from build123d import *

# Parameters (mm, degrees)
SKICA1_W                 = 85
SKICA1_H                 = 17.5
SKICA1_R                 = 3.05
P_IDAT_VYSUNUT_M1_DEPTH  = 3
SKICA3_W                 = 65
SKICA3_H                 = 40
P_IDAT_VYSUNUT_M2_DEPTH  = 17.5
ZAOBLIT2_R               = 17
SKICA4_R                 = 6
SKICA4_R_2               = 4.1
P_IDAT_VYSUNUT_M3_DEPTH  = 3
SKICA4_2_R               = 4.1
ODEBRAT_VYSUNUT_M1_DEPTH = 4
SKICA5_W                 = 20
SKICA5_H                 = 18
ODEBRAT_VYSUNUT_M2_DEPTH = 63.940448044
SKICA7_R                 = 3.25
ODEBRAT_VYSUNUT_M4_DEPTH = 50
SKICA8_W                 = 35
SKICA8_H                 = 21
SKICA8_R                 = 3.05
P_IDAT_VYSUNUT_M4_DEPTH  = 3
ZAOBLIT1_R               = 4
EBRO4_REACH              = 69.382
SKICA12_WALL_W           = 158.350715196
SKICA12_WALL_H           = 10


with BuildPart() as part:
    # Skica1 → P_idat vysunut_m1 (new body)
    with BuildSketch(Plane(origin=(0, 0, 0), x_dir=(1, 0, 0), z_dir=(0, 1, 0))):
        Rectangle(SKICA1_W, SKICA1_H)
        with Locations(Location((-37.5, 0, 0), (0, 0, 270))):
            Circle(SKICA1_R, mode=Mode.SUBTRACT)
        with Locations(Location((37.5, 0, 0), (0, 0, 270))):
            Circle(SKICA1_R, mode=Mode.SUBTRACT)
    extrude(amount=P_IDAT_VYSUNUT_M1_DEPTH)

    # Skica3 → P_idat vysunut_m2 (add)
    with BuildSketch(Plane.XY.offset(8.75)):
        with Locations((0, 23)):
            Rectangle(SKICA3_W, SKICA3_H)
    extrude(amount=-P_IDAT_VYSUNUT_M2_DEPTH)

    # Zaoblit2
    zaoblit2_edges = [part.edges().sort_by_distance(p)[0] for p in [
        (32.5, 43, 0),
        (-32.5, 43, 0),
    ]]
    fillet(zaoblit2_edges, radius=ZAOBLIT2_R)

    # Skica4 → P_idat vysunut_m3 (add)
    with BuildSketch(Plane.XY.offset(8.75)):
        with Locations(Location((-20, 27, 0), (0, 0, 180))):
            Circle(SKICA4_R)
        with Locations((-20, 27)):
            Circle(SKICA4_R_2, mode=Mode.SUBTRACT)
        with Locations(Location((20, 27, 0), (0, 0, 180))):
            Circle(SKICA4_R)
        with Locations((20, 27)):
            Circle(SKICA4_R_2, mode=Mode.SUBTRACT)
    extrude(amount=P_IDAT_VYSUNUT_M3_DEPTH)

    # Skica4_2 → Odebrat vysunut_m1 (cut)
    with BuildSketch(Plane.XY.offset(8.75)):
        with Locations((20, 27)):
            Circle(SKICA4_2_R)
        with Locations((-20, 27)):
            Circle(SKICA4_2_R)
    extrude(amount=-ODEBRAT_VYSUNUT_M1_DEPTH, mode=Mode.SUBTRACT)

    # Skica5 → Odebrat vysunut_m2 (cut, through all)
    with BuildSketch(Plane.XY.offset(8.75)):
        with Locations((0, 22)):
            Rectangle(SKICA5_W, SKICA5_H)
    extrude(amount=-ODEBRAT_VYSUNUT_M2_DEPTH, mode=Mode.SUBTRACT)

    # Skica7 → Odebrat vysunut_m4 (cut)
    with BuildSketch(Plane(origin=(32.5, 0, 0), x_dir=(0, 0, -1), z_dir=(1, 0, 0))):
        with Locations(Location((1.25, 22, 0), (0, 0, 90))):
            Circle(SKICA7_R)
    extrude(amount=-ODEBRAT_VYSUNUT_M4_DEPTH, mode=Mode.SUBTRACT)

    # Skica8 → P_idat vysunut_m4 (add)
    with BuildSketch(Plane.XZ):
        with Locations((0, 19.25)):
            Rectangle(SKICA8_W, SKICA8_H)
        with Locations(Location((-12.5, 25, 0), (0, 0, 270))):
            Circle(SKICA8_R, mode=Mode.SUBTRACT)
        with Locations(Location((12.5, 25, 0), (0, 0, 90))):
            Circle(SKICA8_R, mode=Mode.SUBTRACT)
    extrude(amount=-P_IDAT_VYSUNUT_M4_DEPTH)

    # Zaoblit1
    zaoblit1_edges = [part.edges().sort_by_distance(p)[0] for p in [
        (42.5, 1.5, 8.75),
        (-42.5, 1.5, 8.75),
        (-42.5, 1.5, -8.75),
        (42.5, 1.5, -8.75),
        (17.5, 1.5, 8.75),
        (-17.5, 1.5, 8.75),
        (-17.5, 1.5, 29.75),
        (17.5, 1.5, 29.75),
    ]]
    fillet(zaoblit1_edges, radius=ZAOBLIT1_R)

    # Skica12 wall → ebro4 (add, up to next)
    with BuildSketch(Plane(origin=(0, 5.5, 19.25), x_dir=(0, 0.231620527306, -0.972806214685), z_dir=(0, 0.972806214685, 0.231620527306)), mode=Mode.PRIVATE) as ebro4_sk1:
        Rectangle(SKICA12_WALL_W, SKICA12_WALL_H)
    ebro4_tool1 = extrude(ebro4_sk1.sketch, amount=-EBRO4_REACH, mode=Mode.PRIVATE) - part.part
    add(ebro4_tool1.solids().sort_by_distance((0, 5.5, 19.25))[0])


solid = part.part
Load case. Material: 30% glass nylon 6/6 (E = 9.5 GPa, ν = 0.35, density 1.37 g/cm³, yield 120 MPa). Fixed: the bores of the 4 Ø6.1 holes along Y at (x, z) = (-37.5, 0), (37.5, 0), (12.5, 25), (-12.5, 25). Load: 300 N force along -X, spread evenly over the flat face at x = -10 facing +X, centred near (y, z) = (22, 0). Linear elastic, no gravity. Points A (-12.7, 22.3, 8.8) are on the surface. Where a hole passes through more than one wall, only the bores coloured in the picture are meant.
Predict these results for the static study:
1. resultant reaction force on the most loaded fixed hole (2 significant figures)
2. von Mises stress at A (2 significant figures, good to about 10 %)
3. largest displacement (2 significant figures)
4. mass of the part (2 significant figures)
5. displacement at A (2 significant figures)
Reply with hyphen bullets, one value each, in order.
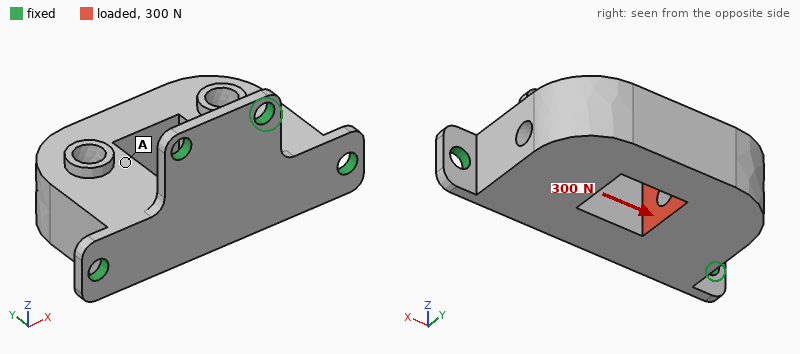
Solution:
- 160 N
- 1.1 MPa
- 14 µm
- 59 g
- 11 µm
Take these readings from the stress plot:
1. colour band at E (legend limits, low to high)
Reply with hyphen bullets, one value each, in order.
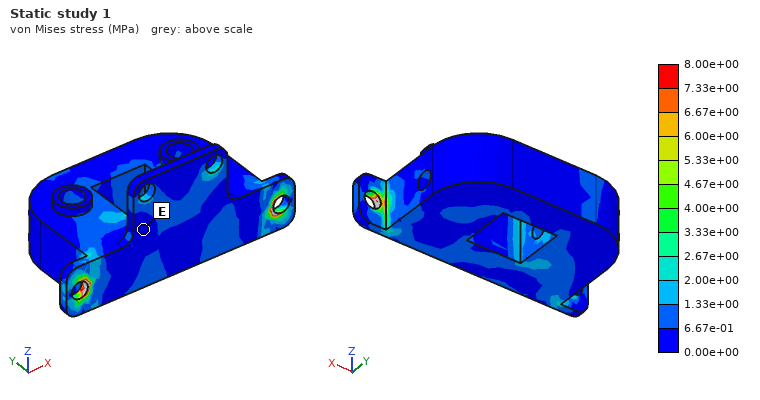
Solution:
- 0.00e+00 to 6.67e-01 MPa
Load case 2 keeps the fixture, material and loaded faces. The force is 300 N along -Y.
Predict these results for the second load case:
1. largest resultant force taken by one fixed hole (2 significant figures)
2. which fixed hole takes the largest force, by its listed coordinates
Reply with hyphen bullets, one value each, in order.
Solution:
- 210 N
- (-37.5, 0)
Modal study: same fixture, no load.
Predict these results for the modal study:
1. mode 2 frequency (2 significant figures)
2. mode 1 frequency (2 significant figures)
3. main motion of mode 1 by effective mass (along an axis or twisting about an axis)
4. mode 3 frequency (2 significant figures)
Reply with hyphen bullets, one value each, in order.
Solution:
- 3700 Hz
- 1100 Hz
- along Z
- 3700 Hz
